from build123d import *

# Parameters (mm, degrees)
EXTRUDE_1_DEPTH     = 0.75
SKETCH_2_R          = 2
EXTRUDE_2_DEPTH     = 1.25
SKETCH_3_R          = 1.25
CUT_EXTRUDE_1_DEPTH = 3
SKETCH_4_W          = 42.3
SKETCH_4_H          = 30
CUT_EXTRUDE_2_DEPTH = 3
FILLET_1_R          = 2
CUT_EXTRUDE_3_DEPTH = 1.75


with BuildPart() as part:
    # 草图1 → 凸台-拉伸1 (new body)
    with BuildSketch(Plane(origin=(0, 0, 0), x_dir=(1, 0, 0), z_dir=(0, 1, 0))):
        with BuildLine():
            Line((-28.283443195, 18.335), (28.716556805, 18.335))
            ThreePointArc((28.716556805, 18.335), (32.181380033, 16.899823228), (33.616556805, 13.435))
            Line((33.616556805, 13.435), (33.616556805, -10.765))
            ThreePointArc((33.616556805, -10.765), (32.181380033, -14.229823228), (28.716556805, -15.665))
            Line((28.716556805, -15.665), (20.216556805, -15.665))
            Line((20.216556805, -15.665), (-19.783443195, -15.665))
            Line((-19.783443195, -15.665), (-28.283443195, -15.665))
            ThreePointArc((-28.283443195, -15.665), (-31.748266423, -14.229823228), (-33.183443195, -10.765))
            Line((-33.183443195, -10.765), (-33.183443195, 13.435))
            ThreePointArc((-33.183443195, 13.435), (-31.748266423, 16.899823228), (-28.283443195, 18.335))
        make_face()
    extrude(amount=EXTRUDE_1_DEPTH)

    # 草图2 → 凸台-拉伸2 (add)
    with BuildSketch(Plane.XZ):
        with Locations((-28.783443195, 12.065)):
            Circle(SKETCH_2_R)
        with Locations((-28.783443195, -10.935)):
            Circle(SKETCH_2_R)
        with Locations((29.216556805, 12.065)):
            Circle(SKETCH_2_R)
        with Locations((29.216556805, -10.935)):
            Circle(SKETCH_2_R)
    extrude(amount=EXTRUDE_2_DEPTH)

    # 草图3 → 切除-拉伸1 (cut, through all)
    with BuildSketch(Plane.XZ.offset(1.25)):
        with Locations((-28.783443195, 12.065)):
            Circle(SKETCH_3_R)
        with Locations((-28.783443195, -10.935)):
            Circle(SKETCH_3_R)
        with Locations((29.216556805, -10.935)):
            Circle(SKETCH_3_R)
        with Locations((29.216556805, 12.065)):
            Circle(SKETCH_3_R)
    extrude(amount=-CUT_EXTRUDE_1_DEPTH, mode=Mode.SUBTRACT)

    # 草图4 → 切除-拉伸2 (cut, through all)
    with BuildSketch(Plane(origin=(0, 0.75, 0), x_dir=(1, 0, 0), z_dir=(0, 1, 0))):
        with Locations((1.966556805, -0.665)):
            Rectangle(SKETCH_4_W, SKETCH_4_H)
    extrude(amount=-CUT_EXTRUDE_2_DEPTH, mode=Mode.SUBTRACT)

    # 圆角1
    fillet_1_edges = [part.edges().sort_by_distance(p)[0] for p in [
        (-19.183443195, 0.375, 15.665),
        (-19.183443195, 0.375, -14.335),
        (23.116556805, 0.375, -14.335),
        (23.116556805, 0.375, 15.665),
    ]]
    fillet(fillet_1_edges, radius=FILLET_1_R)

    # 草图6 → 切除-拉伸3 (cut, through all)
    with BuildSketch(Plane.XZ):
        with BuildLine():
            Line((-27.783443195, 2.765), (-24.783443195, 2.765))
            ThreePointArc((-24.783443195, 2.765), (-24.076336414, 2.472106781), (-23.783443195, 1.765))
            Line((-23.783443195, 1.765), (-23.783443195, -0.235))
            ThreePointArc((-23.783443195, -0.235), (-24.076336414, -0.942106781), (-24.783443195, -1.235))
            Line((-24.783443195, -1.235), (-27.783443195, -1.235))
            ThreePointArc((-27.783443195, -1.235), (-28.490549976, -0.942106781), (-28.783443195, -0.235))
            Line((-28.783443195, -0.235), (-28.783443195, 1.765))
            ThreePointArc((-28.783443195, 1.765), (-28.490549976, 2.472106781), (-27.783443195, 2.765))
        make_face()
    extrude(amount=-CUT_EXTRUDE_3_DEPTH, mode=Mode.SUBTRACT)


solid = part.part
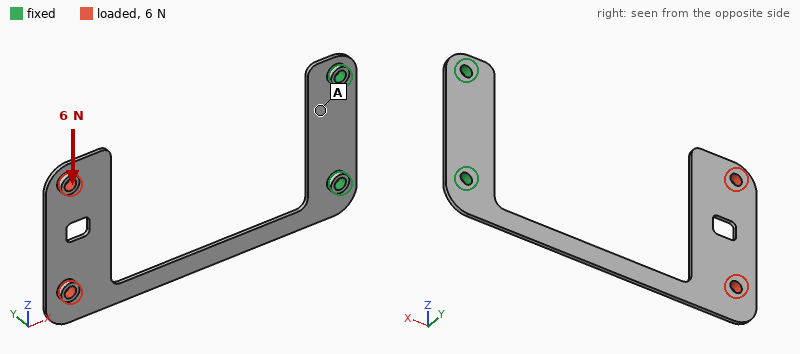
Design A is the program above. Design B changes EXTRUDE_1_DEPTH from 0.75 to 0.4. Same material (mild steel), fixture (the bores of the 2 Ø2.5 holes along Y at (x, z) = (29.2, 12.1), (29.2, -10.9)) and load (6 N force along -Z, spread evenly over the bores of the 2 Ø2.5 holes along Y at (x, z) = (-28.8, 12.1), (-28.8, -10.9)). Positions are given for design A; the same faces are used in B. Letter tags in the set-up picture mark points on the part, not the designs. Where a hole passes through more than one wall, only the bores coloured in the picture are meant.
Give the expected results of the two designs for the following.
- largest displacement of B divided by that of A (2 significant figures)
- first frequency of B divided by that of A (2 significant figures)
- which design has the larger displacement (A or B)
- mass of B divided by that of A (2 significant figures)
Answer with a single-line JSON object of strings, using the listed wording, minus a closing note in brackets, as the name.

{"largest displacement of B divided by that of A": "2.5", "first frequency of B divided by that of A": "0.52", "which design has the larger displacement": "B", "mass of B divided by that of A": "0.56"}
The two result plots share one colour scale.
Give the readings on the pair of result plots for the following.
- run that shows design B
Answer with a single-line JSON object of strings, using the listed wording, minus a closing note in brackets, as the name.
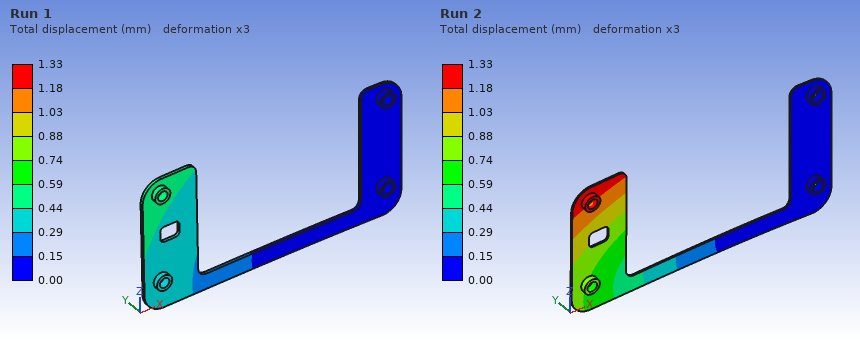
{"run that shows design B": "Run 2"}
